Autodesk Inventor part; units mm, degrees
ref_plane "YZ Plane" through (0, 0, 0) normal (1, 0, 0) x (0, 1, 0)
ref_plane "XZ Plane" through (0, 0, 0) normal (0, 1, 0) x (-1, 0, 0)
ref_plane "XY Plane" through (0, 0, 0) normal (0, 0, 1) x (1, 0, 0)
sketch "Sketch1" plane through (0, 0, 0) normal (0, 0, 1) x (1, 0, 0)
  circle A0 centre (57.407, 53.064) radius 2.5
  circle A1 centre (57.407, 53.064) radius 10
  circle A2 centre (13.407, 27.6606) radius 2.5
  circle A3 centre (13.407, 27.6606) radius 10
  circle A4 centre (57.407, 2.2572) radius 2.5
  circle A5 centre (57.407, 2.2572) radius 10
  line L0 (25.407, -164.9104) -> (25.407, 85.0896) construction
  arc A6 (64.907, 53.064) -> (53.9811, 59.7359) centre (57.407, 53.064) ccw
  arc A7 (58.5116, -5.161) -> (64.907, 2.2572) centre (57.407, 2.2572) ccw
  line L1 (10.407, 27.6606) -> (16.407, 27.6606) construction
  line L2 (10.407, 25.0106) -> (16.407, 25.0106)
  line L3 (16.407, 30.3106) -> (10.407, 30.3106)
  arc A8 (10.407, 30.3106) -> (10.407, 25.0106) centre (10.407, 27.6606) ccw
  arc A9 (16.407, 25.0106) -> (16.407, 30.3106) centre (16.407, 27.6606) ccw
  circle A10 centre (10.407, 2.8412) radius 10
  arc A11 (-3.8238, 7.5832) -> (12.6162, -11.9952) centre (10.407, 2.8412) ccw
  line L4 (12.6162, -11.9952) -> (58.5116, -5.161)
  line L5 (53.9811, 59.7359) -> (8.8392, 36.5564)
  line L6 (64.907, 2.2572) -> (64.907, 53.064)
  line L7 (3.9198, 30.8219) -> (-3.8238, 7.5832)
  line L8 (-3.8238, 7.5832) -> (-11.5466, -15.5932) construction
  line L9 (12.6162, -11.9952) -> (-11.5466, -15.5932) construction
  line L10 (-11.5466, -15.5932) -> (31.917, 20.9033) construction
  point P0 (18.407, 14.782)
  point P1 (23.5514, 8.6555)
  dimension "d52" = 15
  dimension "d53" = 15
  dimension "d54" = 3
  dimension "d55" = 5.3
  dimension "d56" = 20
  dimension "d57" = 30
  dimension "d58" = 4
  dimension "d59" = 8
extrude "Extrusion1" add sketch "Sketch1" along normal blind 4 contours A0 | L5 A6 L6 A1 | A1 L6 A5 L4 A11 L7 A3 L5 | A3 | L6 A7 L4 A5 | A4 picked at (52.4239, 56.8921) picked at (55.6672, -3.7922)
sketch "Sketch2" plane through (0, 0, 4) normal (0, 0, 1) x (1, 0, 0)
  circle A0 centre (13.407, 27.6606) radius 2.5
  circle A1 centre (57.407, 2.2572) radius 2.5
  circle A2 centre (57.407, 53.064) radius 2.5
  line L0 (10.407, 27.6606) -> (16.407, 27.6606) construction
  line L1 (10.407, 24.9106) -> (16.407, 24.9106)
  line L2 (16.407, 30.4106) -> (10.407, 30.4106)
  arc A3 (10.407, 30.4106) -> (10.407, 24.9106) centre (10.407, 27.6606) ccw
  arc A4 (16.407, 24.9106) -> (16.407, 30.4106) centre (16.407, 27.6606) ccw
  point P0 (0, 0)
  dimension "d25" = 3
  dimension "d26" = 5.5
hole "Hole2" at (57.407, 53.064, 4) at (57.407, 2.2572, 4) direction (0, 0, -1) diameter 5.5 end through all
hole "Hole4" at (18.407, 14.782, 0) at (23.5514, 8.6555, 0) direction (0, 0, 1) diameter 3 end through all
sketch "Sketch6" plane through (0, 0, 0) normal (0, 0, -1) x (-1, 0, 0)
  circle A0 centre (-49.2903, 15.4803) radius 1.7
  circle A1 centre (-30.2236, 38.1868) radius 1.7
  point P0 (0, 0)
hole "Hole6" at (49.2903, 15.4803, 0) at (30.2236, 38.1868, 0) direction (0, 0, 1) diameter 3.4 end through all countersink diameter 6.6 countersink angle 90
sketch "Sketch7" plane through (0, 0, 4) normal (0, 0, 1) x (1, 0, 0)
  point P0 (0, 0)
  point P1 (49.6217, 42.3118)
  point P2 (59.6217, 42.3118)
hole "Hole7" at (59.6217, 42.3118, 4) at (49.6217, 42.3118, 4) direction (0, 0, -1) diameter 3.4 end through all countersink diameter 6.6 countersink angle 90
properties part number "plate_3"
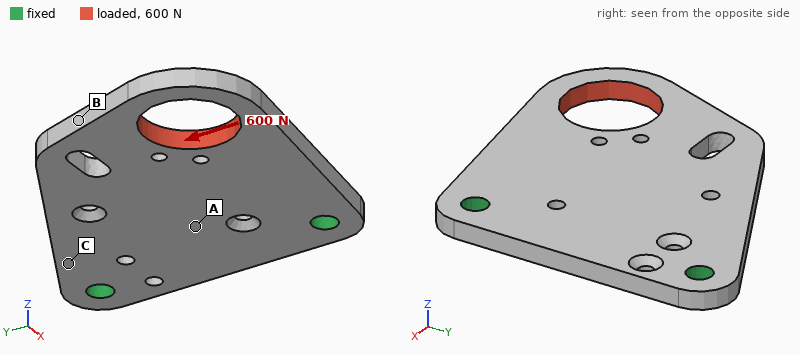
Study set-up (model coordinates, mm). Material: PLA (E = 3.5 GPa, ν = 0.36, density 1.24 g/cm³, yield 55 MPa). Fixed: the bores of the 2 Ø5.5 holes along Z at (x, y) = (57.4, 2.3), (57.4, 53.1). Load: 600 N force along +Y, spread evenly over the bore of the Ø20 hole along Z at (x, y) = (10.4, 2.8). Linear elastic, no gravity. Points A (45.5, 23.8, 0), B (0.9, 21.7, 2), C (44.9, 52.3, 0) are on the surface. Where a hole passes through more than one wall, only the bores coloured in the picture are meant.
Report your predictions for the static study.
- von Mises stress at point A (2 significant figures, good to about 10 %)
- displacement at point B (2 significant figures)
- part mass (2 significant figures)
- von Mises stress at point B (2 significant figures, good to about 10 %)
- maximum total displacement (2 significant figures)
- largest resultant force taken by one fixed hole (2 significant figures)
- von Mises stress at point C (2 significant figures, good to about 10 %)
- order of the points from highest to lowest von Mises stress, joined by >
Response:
3.7 MPa
0.32 mm
16 g
16 MPa
0.45 mm
640 N
9.7 MPa
B > C > A
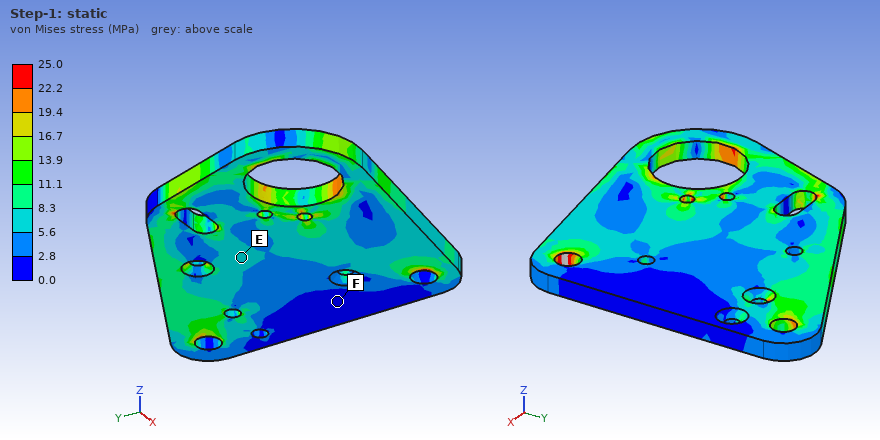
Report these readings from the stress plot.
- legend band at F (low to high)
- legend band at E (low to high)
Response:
0.0 to 2.8 MPa
5.6 to 8.3 MPa
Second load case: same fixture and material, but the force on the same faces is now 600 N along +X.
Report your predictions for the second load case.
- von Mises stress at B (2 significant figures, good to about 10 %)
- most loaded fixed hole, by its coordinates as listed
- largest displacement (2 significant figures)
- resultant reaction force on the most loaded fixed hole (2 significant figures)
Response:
6.1 MPa
(57.4, 2.3)
0.25 mm
590 N
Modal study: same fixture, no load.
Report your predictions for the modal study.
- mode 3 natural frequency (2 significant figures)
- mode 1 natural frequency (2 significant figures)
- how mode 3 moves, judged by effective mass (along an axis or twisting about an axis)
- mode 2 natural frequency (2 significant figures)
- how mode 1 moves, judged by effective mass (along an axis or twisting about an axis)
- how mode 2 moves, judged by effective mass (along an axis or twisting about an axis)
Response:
1700 Hz
370 Hz
along Z
960 Hz
along Z
twisting about X
